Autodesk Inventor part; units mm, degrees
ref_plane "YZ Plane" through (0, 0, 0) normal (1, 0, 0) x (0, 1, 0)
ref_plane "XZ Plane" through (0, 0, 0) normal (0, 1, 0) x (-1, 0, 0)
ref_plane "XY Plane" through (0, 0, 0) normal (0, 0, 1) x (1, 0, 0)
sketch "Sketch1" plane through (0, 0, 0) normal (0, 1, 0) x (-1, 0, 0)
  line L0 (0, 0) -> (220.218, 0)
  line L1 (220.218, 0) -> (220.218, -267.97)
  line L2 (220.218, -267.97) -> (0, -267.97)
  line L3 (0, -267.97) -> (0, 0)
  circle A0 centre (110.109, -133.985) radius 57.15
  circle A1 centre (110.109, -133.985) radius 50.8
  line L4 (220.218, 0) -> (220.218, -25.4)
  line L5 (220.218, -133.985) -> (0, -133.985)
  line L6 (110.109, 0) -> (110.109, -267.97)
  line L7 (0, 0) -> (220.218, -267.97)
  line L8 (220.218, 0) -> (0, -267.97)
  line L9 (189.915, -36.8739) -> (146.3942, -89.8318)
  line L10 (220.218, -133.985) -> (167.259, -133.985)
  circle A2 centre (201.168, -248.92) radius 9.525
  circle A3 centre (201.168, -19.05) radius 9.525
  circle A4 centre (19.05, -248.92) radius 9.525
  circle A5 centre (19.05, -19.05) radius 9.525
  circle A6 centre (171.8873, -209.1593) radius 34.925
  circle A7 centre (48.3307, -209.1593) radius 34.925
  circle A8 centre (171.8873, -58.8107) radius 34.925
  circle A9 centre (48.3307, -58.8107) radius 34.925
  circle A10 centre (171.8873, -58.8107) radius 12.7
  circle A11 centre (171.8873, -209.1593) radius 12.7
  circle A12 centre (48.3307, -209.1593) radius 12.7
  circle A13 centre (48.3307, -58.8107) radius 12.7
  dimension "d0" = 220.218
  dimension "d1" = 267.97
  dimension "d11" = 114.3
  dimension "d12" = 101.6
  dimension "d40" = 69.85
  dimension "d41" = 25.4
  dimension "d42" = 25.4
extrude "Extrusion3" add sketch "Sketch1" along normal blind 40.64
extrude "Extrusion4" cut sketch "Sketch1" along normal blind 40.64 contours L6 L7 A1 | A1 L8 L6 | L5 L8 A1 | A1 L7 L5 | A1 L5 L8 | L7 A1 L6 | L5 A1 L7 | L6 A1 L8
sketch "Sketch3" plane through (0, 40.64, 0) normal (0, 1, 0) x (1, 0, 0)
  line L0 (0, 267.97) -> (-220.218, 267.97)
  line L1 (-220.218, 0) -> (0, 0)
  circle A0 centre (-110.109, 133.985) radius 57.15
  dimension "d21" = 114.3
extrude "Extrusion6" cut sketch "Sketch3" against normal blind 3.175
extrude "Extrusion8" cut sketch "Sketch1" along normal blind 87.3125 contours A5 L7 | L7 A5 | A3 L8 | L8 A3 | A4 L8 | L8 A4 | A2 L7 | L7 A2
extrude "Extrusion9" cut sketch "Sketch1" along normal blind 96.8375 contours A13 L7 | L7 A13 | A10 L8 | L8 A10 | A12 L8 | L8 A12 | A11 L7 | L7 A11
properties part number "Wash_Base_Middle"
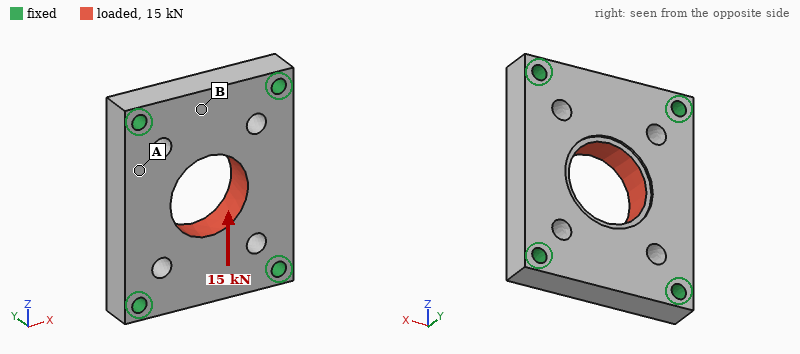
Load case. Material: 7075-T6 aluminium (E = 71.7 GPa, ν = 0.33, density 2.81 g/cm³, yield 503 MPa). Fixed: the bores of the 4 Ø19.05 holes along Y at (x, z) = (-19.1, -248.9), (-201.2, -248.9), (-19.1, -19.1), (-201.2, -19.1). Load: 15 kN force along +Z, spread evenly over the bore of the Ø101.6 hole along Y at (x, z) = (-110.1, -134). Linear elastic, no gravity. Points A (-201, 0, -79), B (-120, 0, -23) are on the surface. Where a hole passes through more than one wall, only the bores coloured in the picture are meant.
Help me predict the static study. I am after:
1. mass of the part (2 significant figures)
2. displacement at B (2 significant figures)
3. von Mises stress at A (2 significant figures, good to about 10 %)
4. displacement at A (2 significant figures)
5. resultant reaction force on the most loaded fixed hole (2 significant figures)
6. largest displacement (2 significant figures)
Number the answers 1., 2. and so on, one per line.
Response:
1. 5.4 kg
2. 2.9 µm
3. 1.0 MPa
4. 1.2 µm
5. 4.0 kN
6. 3.5 µm
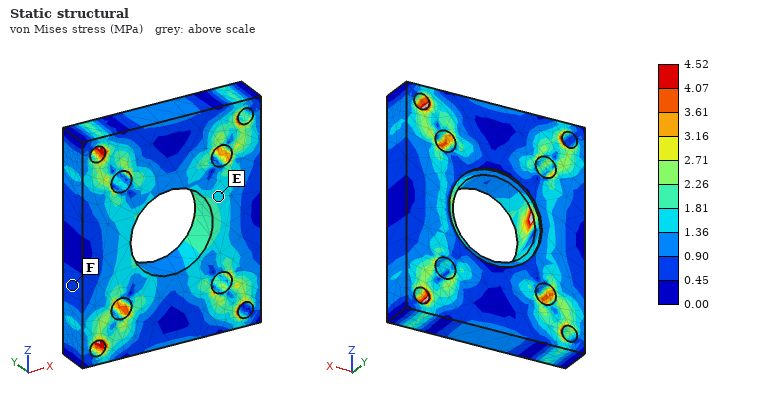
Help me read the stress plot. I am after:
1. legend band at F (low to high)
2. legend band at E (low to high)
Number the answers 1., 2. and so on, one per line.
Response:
1. 0.45 to 0.90 MPa
2. 1.36 to 1.81 MPa
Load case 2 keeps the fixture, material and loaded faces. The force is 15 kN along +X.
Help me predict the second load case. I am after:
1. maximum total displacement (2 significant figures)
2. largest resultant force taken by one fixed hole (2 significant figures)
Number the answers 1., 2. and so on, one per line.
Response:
1. 5.4 µm
2. 4.3 kN
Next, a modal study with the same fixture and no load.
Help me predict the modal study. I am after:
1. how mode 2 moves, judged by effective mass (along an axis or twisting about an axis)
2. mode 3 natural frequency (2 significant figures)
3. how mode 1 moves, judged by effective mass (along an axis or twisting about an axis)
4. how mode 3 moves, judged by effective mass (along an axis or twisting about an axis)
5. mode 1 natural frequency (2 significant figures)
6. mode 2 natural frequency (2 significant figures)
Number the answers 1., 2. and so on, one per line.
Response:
1. twisting about Z
2. 4700 Hz
3. along Y
4. twisting about X
5. 2800 Hz
6. 3700 Hz
